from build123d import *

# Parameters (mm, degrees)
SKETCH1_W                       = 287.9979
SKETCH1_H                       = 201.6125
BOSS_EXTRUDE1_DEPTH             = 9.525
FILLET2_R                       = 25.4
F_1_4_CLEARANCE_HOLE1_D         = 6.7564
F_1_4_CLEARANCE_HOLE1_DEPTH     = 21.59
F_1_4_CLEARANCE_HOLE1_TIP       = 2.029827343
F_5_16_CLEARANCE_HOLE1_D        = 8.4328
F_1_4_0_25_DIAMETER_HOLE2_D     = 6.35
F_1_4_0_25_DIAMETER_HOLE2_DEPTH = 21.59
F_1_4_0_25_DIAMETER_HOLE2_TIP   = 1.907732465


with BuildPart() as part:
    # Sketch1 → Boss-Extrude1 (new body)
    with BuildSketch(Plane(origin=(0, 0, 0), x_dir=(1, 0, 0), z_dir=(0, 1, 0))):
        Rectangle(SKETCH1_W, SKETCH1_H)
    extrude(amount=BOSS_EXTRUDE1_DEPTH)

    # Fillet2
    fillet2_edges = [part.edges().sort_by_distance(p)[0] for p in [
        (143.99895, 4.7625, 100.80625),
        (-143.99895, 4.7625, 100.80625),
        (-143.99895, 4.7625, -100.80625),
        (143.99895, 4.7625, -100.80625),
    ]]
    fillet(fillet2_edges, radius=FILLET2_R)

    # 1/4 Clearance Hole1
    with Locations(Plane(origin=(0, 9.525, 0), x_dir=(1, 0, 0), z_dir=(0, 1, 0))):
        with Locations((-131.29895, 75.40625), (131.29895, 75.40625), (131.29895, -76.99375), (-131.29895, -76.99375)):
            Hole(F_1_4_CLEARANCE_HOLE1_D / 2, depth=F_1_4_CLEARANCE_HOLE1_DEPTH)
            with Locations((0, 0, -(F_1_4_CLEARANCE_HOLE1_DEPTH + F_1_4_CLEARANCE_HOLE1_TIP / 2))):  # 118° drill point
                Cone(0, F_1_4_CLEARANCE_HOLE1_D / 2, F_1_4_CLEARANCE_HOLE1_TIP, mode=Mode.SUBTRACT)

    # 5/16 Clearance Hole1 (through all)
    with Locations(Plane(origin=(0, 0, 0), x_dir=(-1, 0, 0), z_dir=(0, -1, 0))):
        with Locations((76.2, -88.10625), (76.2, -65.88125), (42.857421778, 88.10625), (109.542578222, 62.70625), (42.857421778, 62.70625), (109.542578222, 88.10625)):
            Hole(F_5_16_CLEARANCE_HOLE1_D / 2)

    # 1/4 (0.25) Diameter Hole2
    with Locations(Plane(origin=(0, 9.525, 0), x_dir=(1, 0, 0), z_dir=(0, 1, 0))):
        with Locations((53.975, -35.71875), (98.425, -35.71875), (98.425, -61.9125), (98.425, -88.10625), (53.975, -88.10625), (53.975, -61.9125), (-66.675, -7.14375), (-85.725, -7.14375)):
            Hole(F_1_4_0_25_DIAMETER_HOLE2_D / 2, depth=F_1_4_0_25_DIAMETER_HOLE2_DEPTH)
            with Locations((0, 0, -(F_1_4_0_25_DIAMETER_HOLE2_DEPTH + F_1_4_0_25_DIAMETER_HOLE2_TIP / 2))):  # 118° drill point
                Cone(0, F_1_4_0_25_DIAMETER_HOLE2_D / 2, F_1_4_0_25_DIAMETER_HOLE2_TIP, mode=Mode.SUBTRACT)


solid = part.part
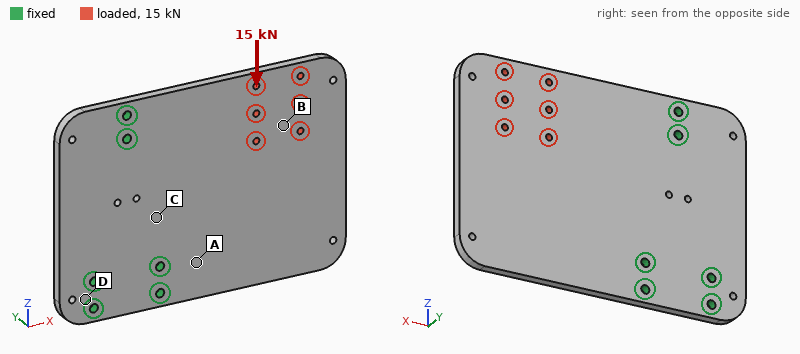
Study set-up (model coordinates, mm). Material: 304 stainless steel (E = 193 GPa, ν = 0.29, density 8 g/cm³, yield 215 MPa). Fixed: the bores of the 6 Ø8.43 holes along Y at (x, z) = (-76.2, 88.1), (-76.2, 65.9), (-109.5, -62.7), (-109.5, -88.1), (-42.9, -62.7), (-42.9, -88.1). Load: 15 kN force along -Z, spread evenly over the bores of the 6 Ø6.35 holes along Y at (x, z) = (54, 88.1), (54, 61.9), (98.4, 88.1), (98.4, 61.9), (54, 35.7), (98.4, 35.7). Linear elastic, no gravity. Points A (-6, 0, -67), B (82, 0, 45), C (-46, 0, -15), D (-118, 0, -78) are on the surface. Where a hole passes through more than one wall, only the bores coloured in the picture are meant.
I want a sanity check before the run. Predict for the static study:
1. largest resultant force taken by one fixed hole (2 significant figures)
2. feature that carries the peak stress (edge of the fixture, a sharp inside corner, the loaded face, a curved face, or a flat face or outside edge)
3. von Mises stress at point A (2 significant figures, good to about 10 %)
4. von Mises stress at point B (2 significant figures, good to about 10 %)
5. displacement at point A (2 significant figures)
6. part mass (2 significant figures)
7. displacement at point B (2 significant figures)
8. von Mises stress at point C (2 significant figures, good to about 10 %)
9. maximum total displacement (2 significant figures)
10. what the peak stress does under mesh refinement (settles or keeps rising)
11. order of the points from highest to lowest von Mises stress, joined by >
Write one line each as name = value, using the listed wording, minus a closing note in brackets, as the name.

largest resultant force taken by one fixed hole = 8.3 kN
feature that carries the peak stress = edge of the fixture
von Mises stress at point A = 20 MPa
von Mises stress at point B = 14 MPa
displacement at point A = 7.7 µm
part mass = 4.3 kg
displacement at point B = 29 µm
von Mises stress at point C = 9.0 MPa
maximum total displacement = 37 µm
what the peak stress does under mesh refinement = keeps rising
order of the points from highest to lowest von Mises stress, joined by > = A > B > C > D
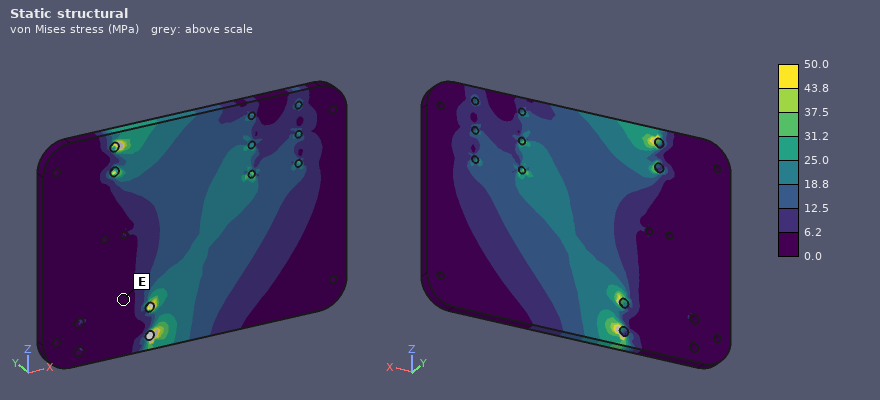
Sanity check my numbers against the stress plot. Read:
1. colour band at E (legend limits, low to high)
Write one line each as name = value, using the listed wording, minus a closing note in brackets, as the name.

colour band at E = 0.0 to 6.2 MPa
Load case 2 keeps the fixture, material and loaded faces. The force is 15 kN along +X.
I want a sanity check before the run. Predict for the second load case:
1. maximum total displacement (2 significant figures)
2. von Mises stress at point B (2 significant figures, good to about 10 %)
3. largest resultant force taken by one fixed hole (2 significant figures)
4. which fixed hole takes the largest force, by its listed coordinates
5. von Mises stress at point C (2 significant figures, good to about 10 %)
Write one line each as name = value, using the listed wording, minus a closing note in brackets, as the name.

maximum total displacement = 24 µm
von Mises stress at point B = 7.3 MPa
largest resultant force taken by one fixed hole = 7.0 kN
which fixed hole takes the largest force, by its listed coordinates = (-76.2, 65.9)
von Mises stress at point C = 4.4 MPa
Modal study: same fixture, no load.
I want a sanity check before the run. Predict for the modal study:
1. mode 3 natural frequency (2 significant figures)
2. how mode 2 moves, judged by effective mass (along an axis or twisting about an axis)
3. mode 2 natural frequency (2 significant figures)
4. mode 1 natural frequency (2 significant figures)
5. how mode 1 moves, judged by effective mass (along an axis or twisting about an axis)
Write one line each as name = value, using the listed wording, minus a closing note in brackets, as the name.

mode 3 natural frequency = 1100 Hz
how mode 2 moves, judged by effective mass = twisting about X
mode 2 natural frequency = 480 Hz
mode 1 natural frequency = 190 Hz
how mode 1 moves, judged by effective mass = along Y
